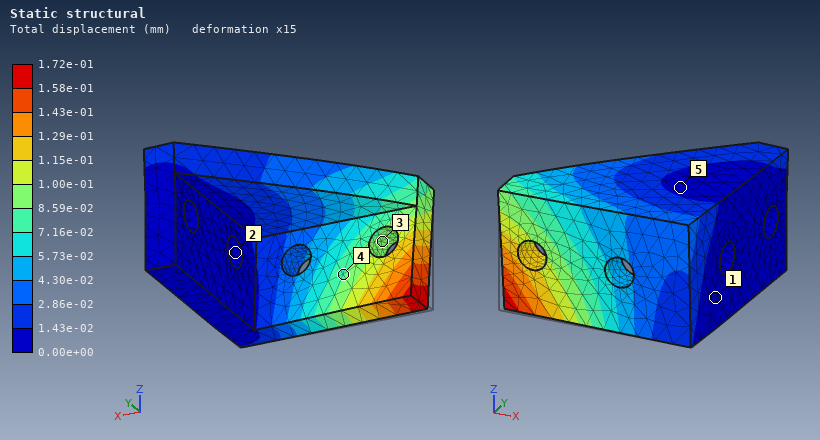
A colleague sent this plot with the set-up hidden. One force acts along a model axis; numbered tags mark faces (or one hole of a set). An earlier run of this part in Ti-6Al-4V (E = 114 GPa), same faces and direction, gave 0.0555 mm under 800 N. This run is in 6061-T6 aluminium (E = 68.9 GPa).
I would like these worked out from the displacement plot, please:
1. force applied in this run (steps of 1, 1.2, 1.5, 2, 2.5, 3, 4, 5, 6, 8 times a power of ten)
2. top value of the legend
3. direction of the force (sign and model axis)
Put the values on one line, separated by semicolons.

1.5 kN; 1.72e-01 mm; +Y
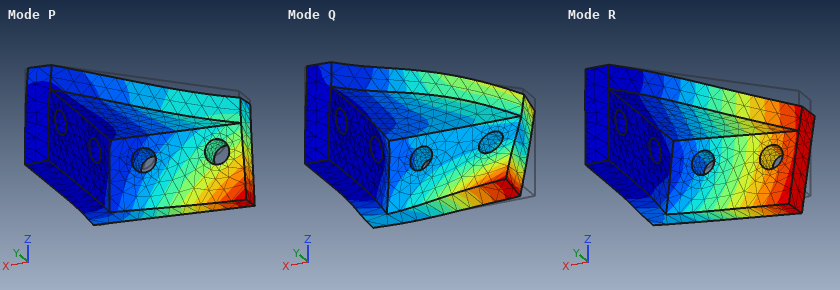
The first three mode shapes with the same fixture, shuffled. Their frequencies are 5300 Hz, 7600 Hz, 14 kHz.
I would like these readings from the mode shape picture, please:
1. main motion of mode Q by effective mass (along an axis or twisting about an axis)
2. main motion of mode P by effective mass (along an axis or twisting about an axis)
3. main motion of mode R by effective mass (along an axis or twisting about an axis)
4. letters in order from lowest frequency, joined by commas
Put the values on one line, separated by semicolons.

along X; along Y; along Z; R, P, Q
